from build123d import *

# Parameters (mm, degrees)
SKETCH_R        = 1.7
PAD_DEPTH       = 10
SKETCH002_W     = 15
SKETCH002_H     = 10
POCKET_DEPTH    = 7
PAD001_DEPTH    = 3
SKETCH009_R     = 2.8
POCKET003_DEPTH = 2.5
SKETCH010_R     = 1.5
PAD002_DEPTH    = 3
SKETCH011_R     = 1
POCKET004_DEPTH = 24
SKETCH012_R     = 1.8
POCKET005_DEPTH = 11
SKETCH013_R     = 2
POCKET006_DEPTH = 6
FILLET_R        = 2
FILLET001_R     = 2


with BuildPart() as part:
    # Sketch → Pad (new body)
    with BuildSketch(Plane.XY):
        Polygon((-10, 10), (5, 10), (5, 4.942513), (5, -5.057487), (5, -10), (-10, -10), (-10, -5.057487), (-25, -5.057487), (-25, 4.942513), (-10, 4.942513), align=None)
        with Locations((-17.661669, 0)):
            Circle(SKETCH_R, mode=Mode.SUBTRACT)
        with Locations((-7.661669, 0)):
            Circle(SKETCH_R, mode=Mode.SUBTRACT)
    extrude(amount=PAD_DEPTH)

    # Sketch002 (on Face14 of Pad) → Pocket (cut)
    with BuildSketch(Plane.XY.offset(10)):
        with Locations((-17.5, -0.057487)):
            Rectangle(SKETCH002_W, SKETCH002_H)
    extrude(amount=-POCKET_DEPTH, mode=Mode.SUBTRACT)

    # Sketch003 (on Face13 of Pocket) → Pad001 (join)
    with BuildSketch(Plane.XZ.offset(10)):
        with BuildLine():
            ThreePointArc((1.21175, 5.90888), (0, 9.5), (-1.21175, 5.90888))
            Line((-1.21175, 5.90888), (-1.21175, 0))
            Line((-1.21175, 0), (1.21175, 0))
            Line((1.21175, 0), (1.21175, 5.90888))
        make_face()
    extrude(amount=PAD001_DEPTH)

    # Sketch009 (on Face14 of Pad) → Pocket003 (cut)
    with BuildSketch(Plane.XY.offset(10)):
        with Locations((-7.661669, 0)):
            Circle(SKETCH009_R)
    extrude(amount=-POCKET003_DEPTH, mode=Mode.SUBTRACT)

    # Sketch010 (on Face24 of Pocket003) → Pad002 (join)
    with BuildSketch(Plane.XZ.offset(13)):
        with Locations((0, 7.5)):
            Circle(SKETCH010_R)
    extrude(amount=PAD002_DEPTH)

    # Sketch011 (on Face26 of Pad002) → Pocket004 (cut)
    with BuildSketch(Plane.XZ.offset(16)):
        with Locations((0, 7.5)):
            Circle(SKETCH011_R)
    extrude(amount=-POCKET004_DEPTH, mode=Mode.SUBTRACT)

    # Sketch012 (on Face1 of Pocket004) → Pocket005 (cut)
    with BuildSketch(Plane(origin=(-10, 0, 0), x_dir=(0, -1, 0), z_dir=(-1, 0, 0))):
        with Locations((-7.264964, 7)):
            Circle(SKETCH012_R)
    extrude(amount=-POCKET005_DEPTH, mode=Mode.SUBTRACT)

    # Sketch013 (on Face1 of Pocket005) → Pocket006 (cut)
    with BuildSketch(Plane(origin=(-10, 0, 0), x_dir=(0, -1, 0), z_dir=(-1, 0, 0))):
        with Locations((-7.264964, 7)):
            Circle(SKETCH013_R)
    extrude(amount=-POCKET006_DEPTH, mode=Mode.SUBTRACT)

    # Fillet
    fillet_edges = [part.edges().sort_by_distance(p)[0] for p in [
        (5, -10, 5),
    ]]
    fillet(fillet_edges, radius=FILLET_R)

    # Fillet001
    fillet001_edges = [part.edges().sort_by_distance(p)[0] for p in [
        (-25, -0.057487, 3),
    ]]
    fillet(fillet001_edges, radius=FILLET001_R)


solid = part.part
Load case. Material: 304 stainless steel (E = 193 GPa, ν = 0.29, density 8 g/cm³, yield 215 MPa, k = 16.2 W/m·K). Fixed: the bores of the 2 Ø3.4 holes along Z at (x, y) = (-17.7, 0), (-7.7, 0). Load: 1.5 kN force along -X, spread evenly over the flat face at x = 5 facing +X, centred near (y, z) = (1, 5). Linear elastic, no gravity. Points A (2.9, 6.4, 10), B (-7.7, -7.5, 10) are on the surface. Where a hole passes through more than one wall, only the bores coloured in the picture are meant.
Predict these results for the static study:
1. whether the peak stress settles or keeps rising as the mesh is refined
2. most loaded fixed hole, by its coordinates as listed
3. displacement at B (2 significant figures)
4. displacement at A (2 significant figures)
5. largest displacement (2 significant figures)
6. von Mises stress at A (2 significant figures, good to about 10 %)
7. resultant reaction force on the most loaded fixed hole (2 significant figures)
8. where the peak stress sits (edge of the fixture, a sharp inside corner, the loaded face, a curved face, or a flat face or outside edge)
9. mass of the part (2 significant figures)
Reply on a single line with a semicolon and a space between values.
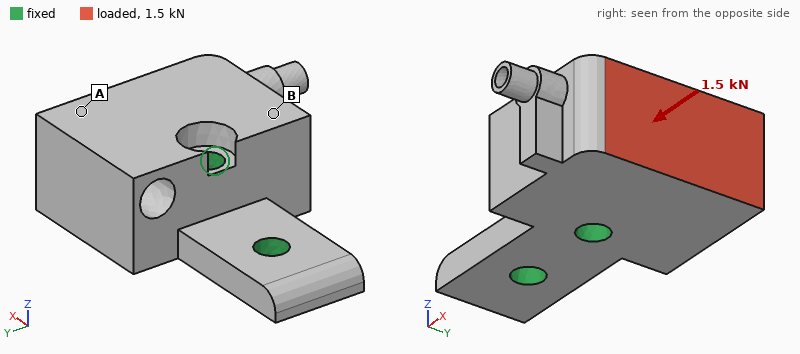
keeps rising; (-7.7, 0); 0.69 µm; 2.4 µm; 3.0 µm; 12 MPa; 1.4 kN; edge of the fixture; 25 g
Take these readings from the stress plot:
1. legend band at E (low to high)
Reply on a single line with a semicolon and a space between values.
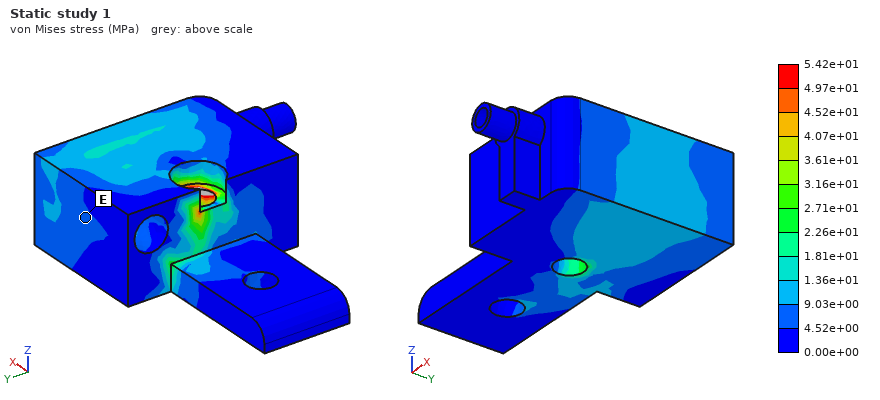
4.52e+00 to 9.03e+00 MPa
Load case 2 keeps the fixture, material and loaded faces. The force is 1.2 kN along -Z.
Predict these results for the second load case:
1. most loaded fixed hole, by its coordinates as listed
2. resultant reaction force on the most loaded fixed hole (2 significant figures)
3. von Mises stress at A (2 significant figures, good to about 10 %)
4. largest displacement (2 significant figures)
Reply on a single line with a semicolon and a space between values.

(-7.7, 0); 1.3 kN; 15 MPa; 12 µm
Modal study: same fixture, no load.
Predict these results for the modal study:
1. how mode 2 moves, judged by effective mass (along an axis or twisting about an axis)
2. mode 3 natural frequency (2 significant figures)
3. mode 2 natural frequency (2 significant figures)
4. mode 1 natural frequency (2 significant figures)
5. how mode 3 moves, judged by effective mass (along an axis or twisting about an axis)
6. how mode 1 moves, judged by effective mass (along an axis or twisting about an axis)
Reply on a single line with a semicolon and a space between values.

along Z; 25 kHz; 21 kHz; 17 kHz; twisting about X; along Y
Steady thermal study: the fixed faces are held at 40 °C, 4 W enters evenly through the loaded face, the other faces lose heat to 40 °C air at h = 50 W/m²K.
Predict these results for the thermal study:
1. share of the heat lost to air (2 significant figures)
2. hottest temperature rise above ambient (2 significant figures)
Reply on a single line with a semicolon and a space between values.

18 %; 21 K
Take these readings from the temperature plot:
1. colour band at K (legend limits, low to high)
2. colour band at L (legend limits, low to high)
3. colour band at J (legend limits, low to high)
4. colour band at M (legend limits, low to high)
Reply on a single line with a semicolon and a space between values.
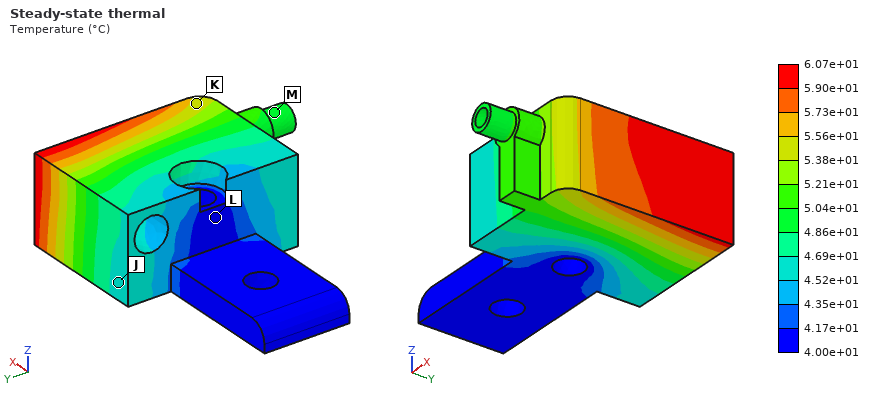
5.38e+01 to 5.56e+01 °C; 4.00e+01 to 4.17e+01 °C; 4.52e+01 to 4.69e+01 °C; 4.86e+01 to 5.04e+01 °C
